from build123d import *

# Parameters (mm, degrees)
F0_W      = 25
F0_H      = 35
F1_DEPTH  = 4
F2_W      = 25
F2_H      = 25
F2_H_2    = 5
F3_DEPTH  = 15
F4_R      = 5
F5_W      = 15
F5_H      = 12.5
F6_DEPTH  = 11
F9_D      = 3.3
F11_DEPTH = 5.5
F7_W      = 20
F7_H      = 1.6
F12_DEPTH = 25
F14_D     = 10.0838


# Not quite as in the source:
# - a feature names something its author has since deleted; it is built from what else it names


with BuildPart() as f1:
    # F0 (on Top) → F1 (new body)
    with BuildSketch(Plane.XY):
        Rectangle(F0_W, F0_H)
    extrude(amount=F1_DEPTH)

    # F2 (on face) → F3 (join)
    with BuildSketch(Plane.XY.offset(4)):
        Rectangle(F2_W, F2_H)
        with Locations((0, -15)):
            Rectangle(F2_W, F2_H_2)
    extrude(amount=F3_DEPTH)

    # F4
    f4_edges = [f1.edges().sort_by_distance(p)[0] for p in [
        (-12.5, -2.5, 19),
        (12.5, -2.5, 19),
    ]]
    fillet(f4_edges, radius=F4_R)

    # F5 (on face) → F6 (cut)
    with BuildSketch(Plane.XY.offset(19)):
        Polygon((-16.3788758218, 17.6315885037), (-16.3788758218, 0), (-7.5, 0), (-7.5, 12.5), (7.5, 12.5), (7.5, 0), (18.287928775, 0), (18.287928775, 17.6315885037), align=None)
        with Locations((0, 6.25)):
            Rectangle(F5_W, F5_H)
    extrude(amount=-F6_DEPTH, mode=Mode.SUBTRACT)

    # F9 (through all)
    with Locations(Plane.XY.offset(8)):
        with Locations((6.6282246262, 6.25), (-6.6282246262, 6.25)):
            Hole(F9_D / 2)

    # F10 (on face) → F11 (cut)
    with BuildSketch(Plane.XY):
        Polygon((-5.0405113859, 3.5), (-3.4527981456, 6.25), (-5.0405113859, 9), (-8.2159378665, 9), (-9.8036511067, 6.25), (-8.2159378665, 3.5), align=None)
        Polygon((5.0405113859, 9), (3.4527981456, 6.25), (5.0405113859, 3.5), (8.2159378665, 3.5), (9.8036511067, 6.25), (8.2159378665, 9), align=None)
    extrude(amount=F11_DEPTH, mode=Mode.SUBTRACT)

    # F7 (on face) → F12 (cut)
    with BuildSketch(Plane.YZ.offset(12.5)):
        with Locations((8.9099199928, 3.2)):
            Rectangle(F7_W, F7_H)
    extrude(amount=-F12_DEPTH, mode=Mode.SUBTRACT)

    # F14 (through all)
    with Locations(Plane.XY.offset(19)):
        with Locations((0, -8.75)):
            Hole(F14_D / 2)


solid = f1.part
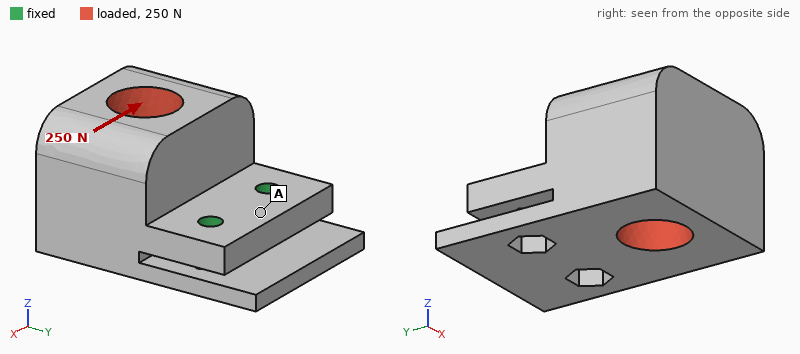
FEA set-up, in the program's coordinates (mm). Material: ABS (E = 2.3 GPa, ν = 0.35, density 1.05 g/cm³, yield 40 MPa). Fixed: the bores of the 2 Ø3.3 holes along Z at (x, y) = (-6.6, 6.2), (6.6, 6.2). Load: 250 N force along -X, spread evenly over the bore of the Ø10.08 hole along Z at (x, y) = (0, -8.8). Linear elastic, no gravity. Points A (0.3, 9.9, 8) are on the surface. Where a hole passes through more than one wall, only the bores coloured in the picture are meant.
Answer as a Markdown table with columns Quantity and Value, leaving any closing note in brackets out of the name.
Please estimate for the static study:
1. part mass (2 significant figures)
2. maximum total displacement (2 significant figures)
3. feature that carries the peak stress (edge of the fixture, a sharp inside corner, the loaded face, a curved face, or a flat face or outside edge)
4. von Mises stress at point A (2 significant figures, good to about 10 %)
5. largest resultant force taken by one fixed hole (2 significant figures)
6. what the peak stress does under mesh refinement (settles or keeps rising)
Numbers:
| Quantity | Value |
|---|---|
| part mass | 9.0 g |
| maximum total displacement | 0.21 mm |
| feature that carries the peak stress | edge of the fixture |
| von Mises stress at point A | 3.4 MPa |
| largest resultant force taken by one fixed hole | 270 N |
| what the peak stress does under mesh refinement | keeps rising |
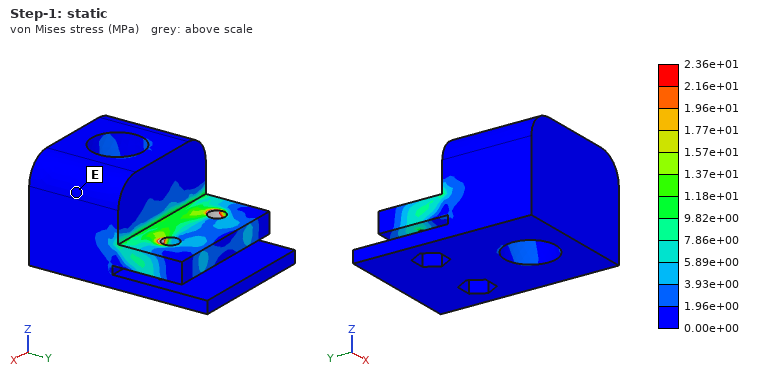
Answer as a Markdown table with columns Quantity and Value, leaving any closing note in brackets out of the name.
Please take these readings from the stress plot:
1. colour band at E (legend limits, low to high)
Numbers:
| Quantity | Value |
|---|---|
| colour band at E | 0.00e+00 to 1.96e+00 MPa |
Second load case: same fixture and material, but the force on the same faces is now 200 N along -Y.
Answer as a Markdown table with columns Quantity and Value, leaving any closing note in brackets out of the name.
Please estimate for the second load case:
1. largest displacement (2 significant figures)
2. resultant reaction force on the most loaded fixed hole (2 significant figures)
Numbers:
| Quantity | Value |
|---|---|
| largest displacement | 0.54 mm |
| resultant reaction force on the most loaded fixed hole | 100 N |
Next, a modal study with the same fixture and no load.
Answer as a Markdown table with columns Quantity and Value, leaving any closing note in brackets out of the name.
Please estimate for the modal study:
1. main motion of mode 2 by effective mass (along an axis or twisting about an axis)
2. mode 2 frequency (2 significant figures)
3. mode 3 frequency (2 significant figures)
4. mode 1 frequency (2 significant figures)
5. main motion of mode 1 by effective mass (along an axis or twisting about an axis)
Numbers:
| Quantity | Value |
|---|---|
| main motion of mode 2 by effective mass | along Z |
| mode 2 frequency | 1300 Hz |
| mode 3 frequency | 2100 Hz |
| mode 1 frequency | 670 Hz |
| main motion of mode 1 by effective mass | along Z |
